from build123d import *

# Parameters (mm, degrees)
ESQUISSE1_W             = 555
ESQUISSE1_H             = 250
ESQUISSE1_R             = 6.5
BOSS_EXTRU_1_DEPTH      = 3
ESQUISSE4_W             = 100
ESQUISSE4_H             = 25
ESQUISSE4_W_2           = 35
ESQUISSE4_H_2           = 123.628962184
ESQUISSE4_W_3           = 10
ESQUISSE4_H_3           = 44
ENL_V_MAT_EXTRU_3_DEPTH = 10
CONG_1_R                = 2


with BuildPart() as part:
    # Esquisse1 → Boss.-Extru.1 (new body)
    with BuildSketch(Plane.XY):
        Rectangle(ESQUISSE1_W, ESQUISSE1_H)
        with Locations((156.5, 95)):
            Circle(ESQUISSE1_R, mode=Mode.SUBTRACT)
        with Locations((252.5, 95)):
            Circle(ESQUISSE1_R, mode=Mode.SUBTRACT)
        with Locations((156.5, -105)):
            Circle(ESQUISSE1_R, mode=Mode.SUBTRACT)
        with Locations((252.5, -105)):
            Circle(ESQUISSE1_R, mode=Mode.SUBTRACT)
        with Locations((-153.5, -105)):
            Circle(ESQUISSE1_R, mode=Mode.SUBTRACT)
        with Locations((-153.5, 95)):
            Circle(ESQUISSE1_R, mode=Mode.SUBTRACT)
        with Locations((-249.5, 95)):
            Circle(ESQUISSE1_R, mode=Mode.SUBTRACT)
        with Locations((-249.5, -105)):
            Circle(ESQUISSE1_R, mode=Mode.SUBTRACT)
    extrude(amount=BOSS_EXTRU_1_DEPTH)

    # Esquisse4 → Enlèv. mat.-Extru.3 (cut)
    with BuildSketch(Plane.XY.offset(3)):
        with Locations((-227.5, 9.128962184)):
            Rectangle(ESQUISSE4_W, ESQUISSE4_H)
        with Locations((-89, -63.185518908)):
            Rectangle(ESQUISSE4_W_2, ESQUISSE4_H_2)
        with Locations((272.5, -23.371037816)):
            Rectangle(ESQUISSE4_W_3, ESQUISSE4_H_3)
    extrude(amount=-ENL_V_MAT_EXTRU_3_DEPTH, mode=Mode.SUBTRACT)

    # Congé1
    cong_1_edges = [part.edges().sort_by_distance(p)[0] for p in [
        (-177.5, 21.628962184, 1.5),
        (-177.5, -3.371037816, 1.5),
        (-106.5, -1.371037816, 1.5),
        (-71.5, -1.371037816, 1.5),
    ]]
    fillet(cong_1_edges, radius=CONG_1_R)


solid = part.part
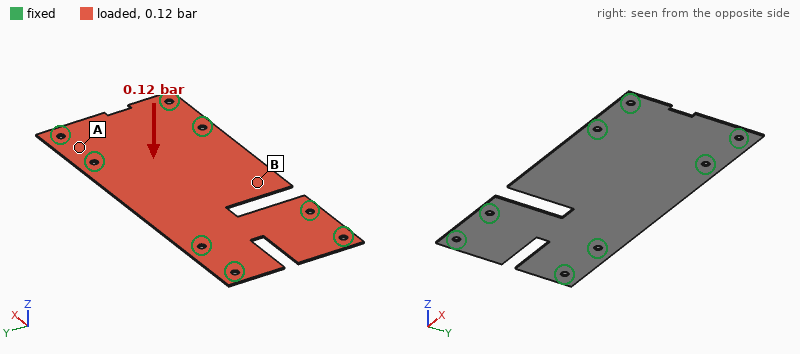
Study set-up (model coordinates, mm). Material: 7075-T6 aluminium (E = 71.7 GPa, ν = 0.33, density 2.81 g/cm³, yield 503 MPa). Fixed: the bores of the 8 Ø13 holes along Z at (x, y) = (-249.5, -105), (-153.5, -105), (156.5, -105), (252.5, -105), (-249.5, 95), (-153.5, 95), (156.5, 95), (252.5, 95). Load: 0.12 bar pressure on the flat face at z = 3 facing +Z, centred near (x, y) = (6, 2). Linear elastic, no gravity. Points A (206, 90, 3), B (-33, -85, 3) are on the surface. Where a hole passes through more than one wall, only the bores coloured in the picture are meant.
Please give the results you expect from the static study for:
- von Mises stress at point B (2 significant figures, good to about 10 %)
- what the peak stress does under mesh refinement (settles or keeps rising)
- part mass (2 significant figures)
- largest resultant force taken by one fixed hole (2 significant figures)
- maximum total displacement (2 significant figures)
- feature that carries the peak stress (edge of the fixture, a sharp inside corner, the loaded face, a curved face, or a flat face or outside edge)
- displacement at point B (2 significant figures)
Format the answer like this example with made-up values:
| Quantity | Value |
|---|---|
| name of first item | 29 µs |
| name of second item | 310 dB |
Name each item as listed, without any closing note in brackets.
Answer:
| Quantity | Value |
|---|---|
| von Mises stress at point B | 31 MPa |
| what the peak stress does under mesh refinement | keeps rising |
| part mass | 1.1 kg |
| largest resultant force taken by one fixed hole | 370 N |
| maximum total displacement | 6.3 mm |
| feature that carries the peak stress | edge of the fixture |
| displacement at point B | 4.8 mm |
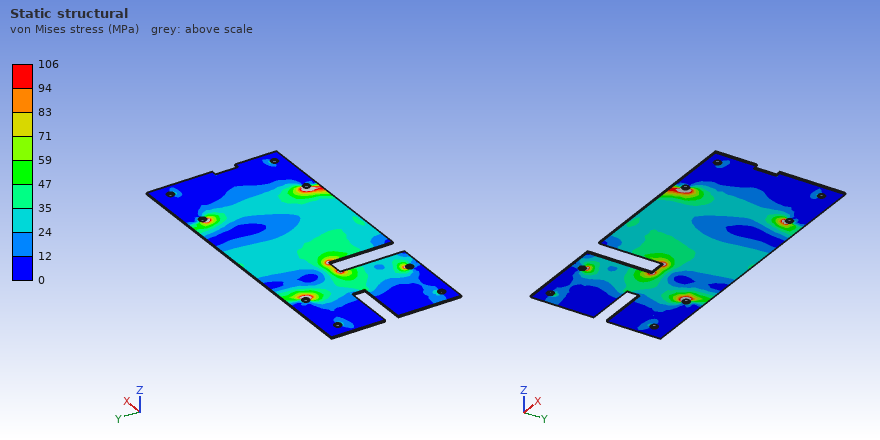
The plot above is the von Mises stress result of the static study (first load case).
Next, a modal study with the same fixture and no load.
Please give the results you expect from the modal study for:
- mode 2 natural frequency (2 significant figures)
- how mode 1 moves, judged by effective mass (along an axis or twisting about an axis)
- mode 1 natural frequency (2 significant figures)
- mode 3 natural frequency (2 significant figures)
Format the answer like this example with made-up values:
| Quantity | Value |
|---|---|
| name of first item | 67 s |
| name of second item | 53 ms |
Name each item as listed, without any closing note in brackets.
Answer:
| Quantity | Value |
|---|---|
| mode 2 natural frequency | 180 Hz |
| how mode 1 moves, judged by effective mass | along Z |
| mode 1 natural frequency | 110 Hz |
| mode 3 natural frequency | 320 Hz |
